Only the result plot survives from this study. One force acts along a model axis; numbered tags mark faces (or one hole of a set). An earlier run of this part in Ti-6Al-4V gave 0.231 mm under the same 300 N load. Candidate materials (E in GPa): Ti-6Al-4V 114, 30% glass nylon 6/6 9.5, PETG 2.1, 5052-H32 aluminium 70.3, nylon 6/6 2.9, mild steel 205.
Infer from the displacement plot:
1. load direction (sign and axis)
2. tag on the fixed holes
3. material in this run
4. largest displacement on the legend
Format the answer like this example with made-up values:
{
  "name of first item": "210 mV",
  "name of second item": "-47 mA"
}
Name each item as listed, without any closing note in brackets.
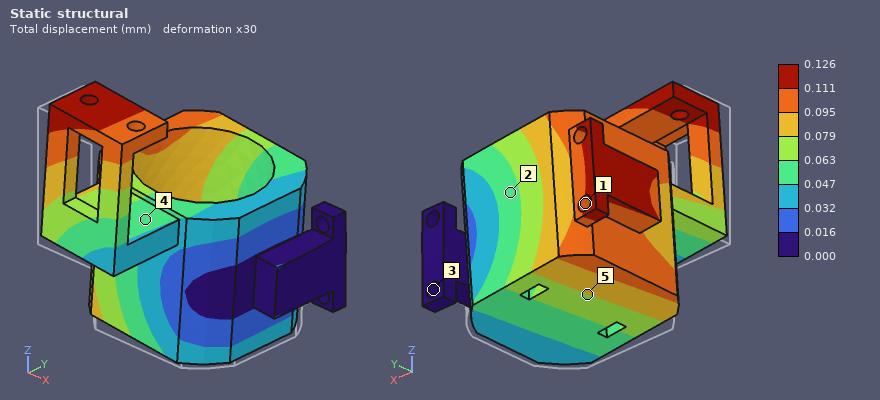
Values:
{
  "load direction": "+Z",
  "tag on the fixed holes": "3",
  "material in this run": "mild steel",
  "largest displacement on the legend": "0.126 mm"
}
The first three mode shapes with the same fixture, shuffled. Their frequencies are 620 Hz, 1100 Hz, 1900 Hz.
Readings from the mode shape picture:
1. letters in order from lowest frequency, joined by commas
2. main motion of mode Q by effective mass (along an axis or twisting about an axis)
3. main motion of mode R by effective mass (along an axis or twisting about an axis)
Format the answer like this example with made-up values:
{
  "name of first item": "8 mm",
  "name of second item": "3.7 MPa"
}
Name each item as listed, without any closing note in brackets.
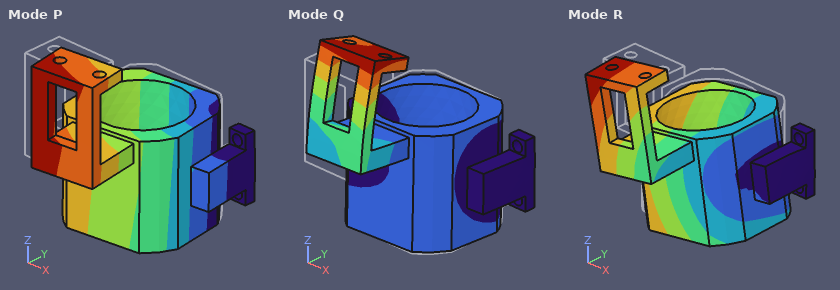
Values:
{
  "letters in order from lowest frequency, joined by commas": "P, R, Q",
  "main motion of mode Q by effective mass": "twisting about X",
  "main motion of mode R by effective mass": "along Z"
}
